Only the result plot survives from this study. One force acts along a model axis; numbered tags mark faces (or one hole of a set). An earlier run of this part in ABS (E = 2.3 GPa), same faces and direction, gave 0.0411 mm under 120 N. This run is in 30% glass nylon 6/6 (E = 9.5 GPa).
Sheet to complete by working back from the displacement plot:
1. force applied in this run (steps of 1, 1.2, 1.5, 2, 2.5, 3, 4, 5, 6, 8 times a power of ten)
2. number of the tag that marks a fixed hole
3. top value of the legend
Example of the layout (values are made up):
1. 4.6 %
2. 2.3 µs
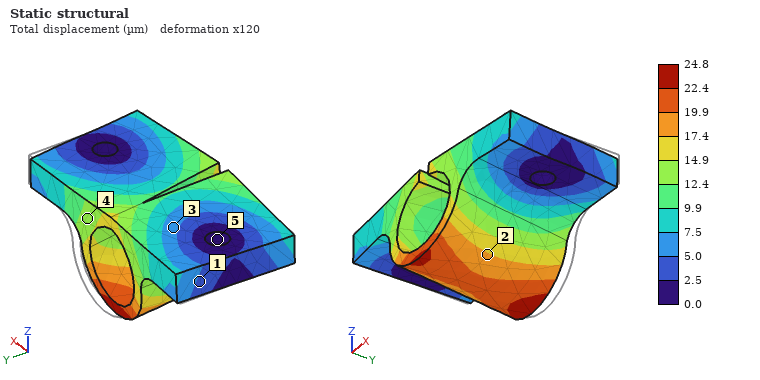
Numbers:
1. 300 N
2. 5
3. 24.8 µm
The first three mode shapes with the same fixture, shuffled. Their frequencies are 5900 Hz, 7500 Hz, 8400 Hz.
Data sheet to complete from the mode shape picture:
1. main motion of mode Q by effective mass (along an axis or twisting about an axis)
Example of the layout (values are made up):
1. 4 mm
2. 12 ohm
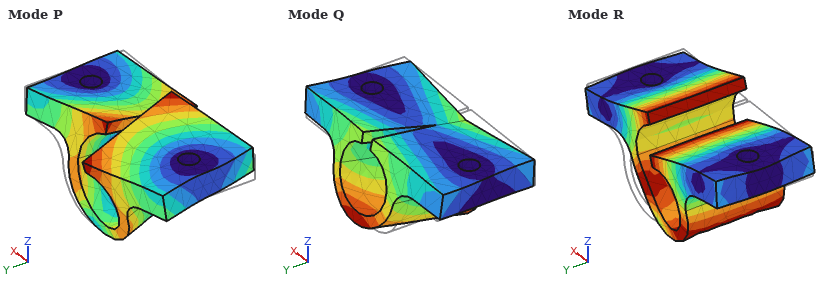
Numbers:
1. along Y
